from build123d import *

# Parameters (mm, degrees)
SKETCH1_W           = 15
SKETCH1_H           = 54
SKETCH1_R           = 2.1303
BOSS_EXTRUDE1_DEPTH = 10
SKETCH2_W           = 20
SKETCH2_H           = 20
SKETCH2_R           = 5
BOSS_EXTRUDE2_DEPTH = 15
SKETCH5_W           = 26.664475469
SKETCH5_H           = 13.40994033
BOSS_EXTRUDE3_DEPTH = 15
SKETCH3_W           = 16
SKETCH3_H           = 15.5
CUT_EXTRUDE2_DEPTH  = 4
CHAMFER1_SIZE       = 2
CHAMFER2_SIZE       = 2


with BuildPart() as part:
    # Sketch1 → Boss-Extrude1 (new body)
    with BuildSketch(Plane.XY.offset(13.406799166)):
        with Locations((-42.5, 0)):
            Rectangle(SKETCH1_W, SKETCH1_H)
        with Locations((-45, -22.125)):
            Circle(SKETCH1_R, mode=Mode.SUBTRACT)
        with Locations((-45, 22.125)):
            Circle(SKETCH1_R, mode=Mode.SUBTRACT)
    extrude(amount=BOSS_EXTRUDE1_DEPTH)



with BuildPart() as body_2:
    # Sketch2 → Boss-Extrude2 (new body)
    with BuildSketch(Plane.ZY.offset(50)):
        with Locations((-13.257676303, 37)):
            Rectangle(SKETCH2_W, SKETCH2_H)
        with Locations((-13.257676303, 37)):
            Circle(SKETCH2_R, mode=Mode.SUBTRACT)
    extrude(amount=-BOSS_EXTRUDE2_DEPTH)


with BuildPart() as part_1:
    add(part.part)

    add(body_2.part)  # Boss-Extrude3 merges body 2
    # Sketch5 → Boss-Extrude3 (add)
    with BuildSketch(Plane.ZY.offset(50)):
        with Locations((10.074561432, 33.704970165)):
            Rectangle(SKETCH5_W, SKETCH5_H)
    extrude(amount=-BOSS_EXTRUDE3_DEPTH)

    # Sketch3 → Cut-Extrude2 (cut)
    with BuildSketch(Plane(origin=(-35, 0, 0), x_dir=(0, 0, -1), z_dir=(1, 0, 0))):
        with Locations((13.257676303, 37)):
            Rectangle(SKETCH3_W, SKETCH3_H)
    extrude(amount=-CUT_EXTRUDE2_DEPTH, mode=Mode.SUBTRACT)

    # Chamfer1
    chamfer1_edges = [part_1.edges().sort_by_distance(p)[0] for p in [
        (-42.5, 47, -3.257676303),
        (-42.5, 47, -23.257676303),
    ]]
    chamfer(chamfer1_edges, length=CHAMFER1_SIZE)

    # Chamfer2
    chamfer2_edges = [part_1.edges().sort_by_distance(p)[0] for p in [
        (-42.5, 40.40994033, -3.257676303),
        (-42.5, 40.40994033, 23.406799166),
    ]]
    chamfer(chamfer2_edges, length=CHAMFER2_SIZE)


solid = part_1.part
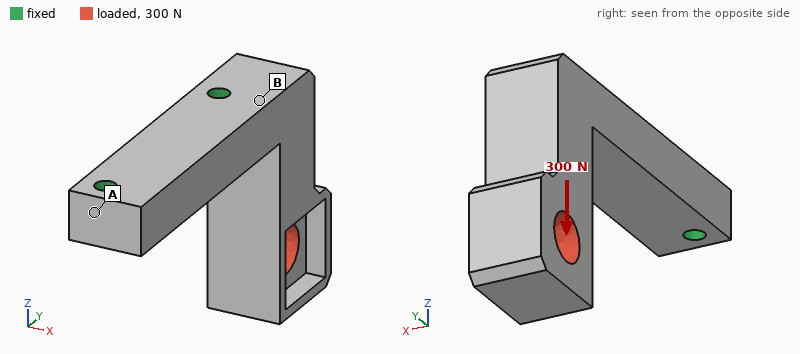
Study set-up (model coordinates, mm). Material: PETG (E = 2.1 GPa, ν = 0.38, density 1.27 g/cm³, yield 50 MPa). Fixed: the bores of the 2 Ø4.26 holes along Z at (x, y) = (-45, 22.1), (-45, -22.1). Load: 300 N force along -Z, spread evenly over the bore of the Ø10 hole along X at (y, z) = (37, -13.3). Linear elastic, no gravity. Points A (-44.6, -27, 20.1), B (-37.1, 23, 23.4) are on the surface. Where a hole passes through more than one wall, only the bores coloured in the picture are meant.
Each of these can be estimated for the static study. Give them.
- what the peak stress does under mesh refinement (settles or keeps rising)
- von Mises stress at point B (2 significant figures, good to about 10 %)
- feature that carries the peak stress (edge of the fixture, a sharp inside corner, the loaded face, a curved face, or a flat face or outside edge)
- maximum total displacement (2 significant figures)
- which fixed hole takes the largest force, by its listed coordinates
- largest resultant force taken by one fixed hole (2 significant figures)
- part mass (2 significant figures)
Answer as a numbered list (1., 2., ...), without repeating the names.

1. keeps rising
2. 7.4 MPa
3. edge of the fixture
4. 0.72 mm
5. (-45, 22.1)
6. 310 N
7. 22 g
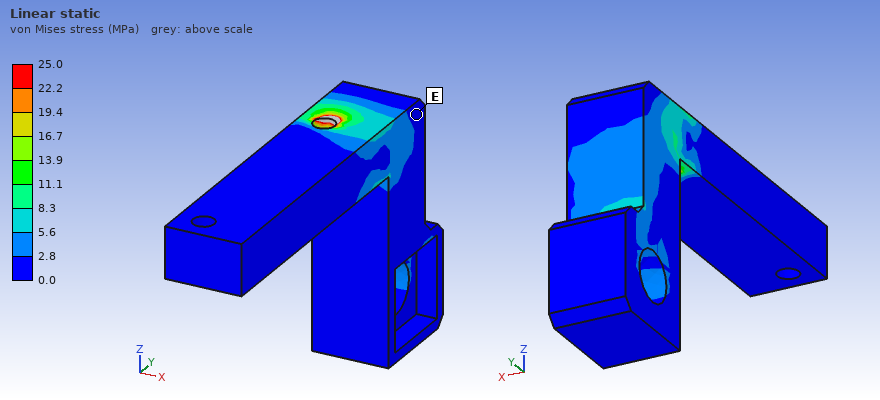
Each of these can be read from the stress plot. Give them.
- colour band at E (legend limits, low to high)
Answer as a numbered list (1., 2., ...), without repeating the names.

1. 0.0 to 2.8 MPa
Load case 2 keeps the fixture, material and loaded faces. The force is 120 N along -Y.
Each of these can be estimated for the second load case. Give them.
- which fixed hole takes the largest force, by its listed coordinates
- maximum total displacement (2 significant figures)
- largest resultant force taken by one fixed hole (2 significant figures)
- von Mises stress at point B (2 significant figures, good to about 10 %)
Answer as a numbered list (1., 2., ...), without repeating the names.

1. (-45, 22.1)
2. 0.93 mm
3. 120 N
4. 7.9 MPa
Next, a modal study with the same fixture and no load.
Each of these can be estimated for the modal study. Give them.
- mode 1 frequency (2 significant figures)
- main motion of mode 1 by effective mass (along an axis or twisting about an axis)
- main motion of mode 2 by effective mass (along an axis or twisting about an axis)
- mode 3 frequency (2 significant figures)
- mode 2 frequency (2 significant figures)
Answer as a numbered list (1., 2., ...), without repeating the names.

1. 830 Hz
2. along Y
3. along X
4. 2600 Hz
5. 880 Hz
